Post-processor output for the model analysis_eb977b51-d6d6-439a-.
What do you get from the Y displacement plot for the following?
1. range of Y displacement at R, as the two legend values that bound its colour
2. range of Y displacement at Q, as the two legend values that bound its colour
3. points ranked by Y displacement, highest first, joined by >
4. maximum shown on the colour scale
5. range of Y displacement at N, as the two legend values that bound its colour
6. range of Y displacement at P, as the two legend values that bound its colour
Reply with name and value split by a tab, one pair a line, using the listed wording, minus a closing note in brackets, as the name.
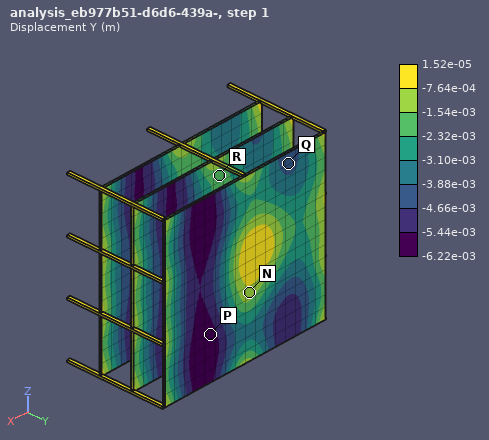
range of Y displacement at R, as the two legend values that bound its colour	-2.32e-03 to -1.54e-03 m
range of Y displacement at Q, as the two legend values that bound its colour	-4.66e-03 to -3.88e-03 m
points ranked by Y displacement, highest first, joined by >	N > R > Q > P
maximum shown on the colour scale	1.52e-05 m
range of Y displacement at N, as the two legend values that bound its colour	-1.54e-03 to -7.64e-04 m
range of Y displacement at P, as the two legend values that bound its colour	-6.22e-03 to -5.44e-03 m
